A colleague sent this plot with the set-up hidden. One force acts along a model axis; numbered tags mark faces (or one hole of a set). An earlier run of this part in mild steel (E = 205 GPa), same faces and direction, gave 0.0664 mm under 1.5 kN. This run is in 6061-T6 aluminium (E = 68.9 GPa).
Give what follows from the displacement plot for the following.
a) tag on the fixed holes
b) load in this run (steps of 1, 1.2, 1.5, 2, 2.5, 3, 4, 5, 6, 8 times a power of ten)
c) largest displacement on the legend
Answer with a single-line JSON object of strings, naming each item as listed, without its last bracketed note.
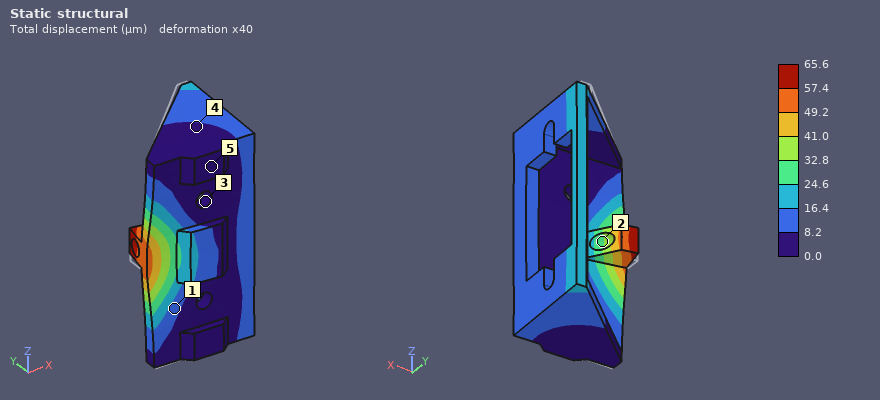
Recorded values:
{"tag on the fixed holes": "3", "load in this run": "500 N", "largest displacement on the legend": "65.6 µm"}
